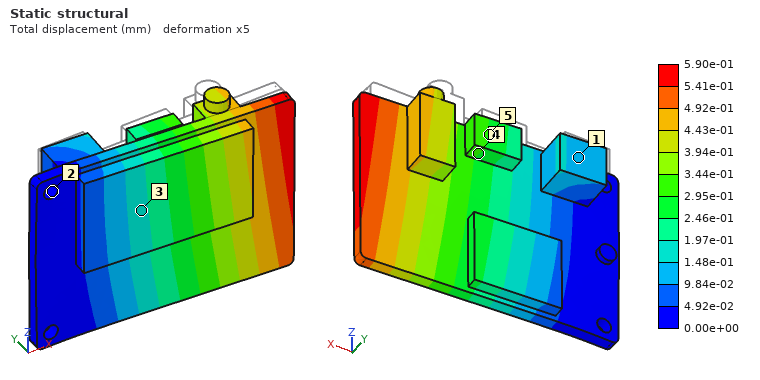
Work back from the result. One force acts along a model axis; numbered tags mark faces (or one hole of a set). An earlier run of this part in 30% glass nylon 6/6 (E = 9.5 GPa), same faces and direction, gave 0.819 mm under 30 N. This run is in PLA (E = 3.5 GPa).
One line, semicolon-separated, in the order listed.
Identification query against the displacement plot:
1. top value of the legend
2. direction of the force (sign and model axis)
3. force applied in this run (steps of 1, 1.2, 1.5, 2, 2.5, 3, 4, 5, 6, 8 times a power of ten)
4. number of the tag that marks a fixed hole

5.90e-01 mm; -Y; 8 N; 2
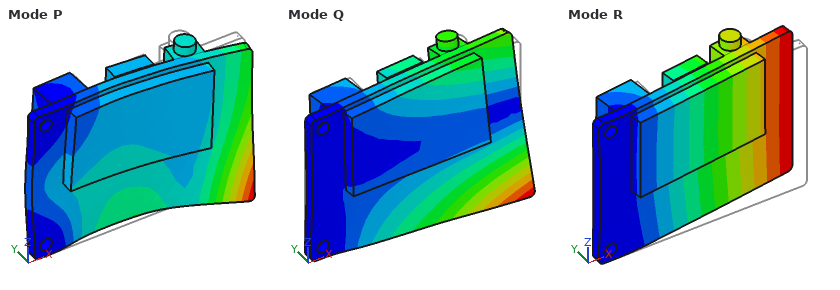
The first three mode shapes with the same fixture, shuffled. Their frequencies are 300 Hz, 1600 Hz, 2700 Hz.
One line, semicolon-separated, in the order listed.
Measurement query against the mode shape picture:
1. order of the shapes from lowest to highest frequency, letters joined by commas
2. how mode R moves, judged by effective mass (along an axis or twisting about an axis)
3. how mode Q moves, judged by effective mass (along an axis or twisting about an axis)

R, Q, P; along Y; twisting about X
